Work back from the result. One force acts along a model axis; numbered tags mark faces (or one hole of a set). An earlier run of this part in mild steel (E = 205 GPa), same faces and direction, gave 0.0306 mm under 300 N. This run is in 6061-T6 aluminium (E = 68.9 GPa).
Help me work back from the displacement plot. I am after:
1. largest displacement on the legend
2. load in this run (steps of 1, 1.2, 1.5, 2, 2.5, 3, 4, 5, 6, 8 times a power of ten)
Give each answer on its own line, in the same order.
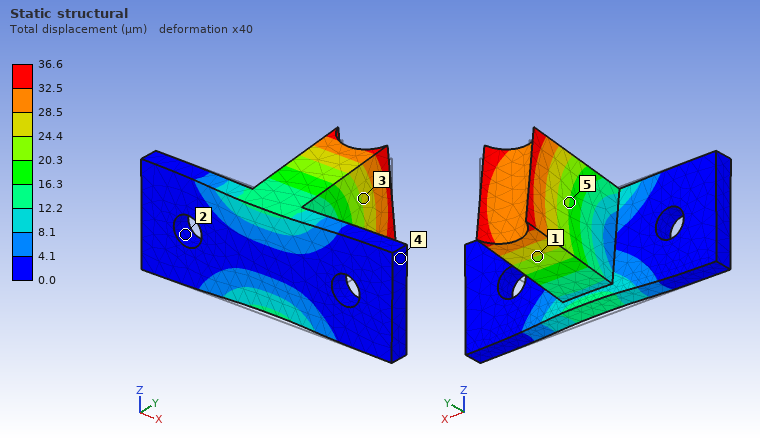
36.6 µm
120 N
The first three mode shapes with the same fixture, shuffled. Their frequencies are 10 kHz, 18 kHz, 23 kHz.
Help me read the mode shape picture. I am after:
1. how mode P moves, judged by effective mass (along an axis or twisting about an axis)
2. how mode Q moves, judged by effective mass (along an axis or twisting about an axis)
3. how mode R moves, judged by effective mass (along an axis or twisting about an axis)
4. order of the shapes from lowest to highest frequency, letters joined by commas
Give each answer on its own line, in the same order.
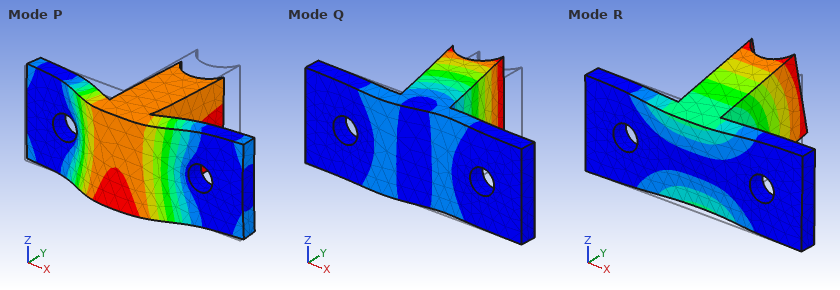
along Y
along X
along Z
R, Q, P
